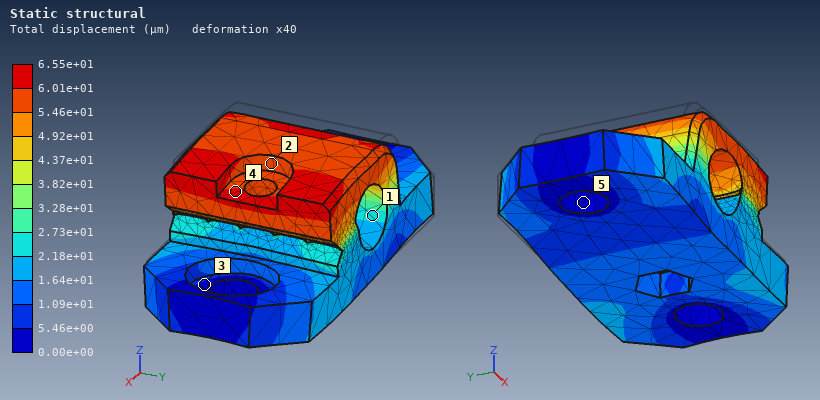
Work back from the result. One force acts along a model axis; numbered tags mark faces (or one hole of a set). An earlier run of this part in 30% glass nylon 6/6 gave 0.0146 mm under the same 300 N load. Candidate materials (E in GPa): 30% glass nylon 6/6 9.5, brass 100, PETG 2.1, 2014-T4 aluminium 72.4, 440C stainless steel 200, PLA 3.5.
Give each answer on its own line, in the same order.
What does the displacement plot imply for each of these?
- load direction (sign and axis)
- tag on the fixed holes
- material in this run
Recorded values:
+X
5
PETG
